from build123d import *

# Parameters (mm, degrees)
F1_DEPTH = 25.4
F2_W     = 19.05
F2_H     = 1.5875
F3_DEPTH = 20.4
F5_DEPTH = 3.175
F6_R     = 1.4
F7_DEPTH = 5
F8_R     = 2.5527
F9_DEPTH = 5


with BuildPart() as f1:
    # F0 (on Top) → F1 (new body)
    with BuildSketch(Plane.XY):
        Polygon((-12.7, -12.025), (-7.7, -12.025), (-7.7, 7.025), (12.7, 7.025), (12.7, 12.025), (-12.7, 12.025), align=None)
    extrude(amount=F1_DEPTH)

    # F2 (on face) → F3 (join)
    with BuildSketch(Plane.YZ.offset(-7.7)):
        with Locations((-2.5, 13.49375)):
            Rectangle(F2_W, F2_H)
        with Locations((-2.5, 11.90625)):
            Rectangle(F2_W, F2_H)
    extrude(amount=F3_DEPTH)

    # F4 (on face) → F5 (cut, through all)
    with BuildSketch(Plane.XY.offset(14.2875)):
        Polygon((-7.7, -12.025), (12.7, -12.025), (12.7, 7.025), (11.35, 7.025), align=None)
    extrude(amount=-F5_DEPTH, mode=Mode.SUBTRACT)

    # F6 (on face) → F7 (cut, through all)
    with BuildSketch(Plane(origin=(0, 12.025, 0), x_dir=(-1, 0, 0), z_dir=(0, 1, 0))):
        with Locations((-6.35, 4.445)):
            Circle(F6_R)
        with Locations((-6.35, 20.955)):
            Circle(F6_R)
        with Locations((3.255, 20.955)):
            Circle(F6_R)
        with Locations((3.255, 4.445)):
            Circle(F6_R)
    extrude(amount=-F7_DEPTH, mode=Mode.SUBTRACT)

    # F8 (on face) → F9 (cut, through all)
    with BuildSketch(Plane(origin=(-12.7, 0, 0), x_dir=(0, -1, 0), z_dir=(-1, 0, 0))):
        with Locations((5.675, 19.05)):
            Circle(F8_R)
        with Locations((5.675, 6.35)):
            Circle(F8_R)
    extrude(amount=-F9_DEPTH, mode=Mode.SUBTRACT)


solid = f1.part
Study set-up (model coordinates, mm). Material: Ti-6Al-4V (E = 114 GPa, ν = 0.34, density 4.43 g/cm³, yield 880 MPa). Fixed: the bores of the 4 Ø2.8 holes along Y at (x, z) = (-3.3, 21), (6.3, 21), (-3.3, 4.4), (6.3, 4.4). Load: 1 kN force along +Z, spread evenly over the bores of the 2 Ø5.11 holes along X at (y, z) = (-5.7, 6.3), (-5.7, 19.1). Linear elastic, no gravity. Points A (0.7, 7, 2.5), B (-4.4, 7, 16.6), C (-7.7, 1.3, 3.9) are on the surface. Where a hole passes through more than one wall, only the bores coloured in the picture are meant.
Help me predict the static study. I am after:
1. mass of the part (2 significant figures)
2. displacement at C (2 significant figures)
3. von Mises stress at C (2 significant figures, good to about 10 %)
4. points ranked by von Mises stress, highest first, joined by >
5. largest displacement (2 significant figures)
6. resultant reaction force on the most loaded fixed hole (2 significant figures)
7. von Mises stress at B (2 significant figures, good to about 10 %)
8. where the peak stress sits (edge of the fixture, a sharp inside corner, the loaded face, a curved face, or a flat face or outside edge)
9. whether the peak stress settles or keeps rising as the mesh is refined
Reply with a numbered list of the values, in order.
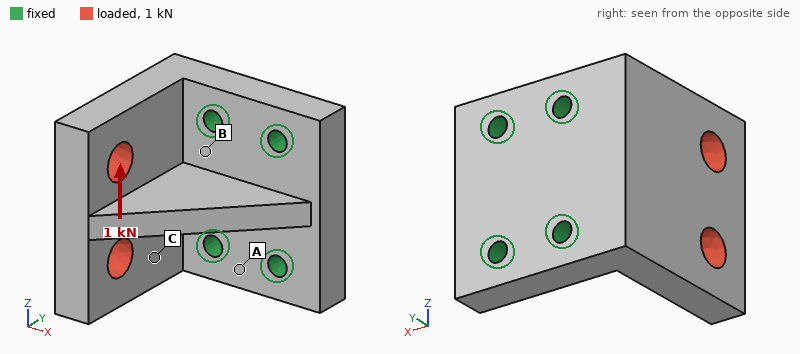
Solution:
1. 26 g
2. 9.2 µm
3. 21 MPa
4. B > C > A
5. 21 µm
6. 1.0 kN
7. 35 MPa
8. edge of the fixture
9. keeps rising
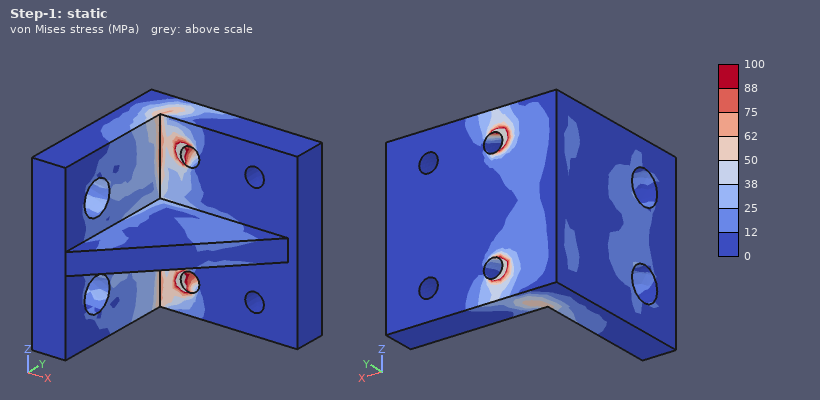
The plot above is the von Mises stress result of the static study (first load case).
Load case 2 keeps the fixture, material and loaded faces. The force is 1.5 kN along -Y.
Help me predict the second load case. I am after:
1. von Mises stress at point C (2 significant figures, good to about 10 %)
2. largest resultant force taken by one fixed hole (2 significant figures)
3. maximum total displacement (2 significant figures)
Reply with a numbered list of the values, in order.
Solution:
1. 18 MPa
2. 940 N
3. 16 µm
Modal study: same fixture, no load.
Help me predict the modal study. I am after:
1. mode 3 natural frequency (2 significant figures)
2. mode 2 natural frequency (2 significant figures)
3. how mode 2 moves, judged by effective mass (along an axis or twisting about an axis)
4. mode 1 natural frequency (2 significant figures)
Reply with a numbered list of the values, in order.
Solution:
1. 18 kHz
2. 13 kHz
3. along Z
4. 12 kHz
